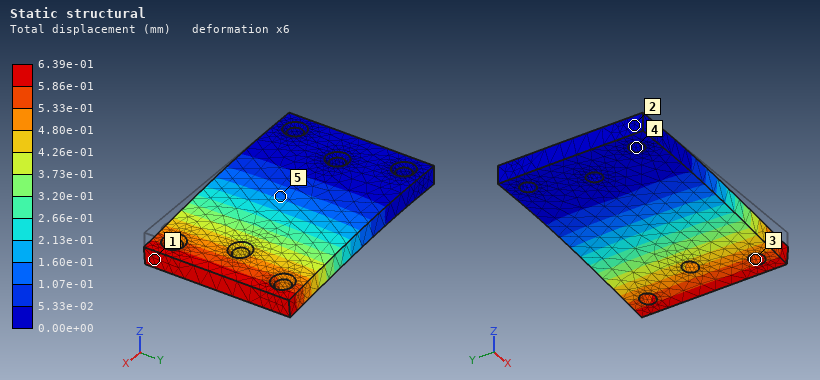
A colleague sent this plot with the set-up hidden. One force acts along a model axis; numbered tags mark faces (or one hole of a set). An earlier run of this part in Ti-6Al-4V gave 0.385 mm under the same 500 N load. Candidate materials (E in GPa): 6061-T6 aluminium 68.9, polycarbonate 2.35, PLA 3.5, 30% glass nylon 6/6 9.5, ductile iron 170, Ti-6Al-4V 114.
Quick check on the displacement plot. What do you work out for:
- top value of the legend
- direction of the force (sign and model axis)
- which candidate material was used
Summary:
6.39e-01 mm
-Z
6061-T6 aluminium
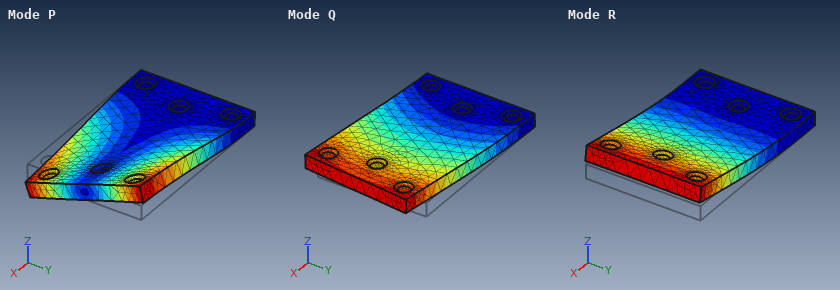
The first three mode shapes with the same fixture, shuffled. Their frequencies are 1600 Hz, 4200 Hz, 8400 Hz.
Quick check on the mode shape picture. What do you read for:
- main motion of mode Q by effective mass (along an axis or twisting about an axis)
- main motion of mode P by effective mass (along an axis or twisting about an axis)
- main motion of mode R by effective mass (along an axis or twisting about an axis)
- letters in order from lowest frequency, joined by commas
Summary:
along Y
twisting about X
along Z
R, P, Q
